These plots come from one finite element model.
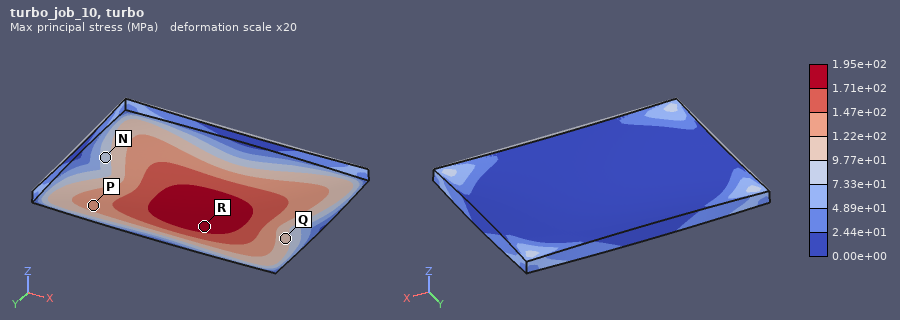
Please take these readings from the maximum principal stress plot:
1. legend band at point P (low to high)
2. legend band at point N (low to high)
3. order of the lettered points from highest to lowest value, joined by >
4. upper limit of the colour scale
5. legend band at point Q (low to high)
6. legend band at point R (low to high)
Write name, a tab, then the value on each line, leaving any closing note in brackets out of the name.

legend band at point P	1.22e+02 to 1.47e+02 MPa
legend band at point N	7.33e+01 to 9.77e+01 MPa
order of the lettered points from highest to lowest value, joined by >	R > P > Q > N
upper limit of the colour scale	1.95e+02 MPa
legend band at point Q	9.77e+01 to 1.22e+02 MPa
legend band at point R	1.71e+02 to 1.95e+02 MPa
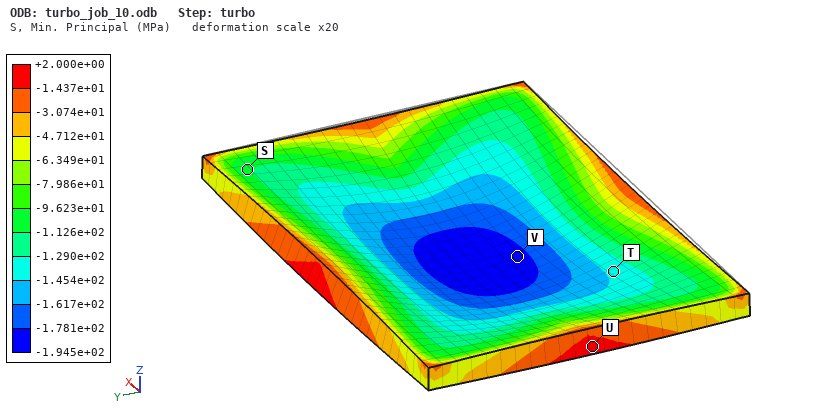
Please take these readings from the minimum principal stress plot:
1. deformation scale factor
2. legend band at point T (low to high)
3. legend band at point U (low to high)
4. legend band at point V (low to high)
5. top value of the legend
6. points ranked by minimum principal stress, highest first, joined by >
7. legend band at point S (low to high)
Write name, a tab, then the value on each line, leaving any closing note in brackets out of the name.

deformation scale factor	20
legend band at point T	-1.454e+02 to -1.290e+02 MPa
legend band at point U	-1.437e+01 to +2.000e+00 MPa
legend band at point V	-1.945e+02 to -1.781e+02 MPa
top value of the legend	+2.000e+00 MPa
points ranked by minimum principal stress, highest first, joined by >	U > S > T > V
legend band at point S	-1.126e+02 to -9.623e+01 MPa
